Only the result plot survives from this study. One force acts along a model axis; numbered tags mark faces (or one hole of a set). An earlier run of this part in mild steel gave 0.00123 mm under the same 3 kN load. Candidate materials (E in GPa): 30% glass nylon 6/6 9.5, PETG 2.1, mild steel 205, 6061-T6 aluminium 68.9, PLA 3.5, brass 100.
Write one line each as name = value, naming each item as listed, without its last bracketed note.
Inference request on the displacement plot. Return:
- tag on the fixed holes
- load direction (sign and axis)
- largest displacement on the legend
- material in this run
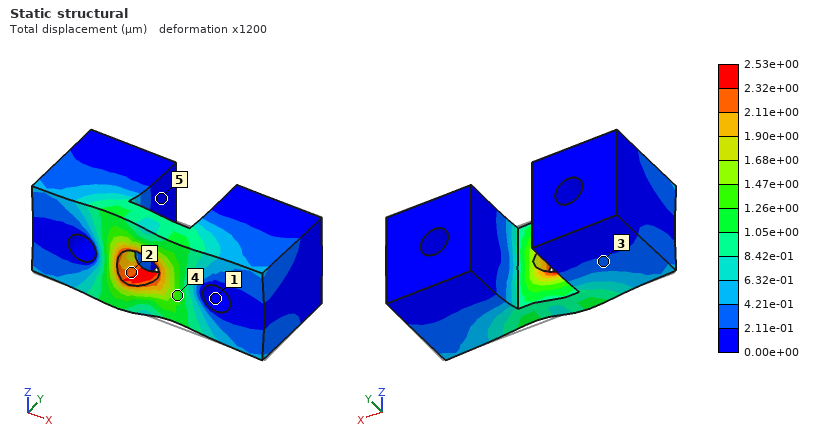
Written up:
tag on the fixed holes = 1
load direction = -X
largest displacement on the legend = 2.53e+00 µm
material in this run = brass
